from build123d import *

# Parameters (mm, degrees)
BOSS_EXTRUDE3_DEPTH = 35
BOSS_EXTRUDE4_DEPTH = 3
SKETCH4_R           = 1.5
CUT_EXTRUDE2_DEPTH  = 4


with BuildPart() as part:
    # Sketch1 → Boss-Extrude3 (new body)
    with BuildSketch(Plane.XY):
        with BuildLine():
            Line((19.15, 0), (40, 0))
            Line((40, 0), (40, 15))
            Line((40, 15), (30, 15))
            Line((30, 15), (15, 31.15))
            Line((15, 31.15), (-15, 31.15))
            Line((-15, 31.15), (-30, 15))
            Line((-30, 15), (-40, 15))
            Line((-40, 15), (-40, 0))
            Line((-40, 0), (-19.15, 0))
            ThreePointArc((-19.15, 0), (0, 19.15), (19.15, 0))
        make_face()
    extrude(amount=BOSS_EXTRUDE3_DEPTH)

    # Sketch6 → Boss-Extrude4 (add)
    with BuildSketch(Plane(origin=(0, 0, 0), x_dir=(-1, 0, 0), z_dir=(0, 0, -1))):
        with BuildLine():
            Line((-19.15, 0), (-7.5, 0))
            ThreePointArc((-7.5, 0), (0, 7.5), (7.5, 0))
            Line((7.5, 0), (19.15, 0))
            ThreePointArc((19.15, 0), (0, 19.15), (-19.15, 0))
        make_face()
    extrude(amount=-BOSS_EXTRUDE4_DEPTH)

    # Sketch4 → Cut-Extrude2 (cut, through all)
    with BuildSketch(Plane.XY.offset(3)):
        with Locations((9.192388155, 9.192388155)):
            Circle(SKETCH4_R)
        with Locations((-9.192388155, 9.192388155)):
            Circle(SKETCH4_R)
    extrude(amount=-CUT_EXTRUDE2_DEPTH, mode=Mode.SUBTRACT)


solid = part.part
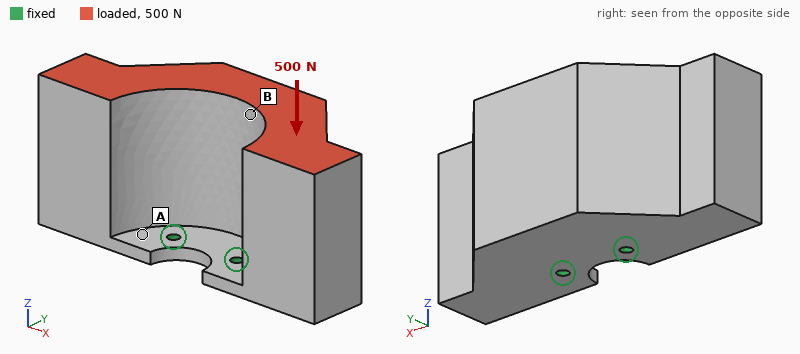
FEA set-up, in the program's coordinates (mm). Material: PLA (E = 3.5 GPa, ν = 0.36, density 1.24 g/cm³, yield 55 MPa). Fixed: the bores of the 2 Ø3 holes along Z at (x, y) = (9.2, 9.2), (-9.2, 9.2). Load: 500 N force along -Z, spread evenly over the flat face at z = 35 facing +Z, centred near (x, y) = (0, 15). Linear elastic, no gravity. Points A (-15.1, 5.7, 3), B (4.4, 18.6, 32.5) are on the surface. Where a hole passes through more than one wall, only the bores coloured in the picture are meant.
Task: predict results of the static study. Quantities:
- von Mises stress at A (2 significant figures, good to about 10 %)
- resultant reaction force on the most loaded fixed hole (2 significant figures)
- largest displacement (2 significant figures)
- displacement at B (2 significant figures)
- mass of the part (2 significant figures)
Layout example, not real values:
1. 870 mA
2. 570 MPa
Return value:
1. 11 MPa
2. 250 N
3. 1.0 mm
4. 0.84 mm
5. 60 g
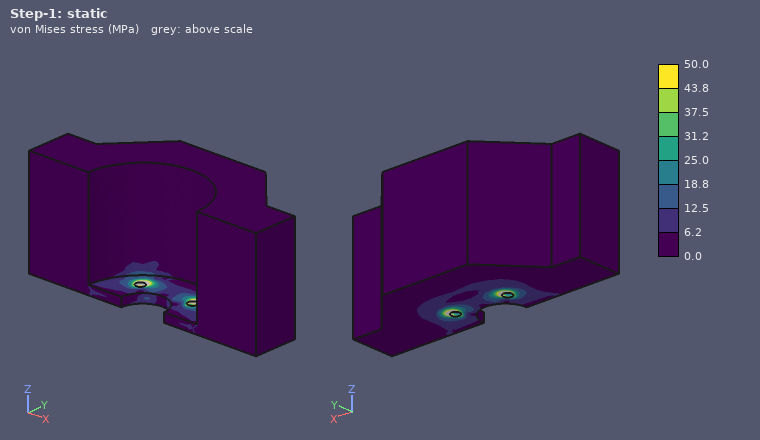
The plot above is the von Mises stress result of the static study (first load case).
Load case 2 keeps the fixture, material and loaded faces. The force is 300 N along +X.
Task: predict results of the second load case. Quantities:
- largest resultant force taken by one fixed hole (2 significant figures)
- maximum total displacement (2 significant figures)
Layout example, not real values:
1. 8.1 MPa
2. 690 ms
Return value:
1. 450 N
2. 1.0 mm
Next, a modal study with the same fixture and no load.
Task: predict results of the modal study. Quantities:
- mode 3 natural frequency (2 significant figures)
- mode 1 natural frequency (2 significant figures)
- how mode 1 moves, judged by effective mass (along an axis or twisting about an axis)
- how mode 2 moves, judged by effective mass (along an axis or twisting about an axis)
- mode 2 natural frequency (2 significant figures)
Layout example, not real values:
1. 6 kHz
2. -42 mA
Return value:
1. 1000 Hz
2. 270 Hz
3. along Y
4. along X
5. 530 Hz
